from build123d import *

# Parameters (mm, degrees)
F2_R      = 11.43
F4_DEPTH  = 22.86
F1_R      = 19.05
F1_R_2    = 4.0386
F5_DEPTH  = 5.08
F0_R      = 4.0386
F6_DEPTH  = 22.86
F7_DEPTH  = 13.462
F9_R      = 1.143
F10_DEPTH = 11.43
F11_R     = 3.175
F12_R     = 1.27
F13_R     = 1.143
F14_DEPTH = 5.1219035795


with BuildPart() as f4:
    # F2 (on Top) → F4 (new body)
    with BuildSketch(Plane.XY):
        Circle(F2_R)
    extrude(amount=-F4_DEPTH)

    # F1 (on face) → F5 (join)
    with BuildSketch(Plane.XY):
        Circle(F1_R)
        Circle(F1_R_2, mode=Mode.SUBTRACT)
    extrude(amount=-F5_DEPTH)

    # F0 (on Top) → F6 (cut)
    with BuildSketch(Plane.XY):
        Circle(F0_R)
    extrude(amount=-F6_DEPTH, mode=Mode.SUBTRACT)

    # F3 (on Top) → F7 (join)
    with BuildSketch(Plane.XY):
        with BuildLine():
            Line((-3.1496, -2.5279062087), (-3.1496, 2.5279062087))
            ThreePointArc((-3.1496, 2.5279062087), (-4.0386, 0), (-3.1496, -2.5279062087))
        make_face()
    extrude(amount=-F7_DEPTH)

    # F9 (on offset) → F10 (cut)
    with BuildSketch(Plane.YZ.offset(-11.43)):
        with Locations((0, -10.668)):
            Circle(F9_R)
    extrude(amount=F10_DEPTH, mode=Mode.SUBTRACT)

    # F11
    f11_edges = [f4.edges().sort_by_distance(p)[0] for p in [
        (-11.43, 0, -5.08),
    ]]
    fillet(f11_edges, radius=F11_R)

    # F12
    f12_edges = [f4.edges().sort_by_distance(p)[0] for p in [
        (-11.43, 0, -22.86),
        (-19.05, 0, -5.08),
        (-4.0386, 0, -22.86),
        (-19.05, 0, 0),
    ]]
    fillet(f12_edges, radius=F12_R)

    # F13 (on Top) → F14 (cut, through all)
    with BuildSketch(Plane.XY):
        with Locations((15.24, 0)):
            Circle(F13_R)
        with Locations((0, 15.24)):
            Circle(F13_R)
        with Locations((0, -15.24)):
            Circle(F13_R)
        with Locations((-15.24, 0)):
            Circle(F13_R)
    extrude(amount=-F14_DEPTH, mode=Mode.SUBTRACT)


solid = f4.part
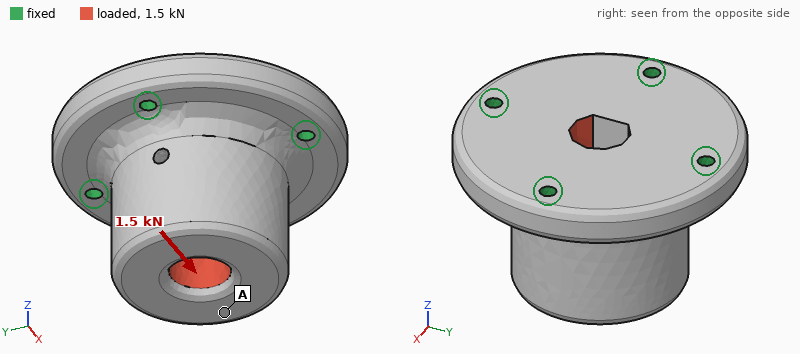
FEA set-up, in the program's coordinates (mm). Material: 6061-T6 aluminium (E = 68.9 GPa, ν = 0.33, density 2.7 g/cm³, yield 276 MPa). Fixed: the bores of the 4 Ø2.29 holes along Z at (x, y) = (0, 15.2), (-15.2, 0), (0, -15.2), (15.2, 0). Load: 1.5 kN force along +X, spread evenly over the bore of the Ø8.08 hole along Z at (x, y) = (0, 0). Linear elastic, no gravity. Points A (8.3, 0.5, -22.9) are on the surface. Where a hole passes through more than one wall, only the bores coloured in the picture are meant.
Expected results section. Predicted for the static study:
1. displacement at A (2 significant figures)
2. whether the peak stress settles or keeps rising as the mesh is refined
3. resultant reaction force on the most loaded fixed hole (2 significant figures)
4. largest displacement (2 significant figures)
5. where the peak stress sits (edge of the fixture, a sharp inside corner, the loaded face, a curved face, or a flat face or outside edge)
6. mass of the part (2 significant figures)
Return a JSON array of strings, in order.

["6.2 µm", "keeps rising", "680 N", "6.4 µm", "edge of the fixture", "32 g"]
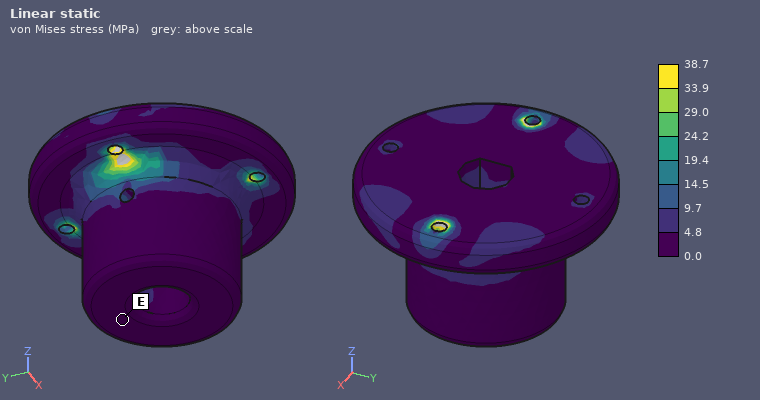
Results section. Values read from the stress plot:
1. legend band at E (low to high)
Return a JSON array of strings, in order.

["0.0 to 4.8 MPa"]
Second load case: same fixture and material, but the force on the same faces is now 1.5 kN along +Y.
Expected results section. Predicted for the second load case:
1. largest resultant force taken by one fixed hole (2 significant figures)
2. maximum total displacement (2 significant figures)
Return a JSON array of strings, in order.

["660 N", "6.3 µm"]
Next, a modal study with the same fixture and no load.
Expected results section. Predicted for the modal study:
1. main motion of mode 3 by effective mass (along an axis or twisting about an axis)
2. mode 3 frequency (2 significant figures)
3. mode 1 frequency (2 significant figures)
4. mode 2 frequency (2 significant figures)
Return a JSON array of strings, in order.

["along Z", "25 kHz", "19 kHz", "19 kHz"]
